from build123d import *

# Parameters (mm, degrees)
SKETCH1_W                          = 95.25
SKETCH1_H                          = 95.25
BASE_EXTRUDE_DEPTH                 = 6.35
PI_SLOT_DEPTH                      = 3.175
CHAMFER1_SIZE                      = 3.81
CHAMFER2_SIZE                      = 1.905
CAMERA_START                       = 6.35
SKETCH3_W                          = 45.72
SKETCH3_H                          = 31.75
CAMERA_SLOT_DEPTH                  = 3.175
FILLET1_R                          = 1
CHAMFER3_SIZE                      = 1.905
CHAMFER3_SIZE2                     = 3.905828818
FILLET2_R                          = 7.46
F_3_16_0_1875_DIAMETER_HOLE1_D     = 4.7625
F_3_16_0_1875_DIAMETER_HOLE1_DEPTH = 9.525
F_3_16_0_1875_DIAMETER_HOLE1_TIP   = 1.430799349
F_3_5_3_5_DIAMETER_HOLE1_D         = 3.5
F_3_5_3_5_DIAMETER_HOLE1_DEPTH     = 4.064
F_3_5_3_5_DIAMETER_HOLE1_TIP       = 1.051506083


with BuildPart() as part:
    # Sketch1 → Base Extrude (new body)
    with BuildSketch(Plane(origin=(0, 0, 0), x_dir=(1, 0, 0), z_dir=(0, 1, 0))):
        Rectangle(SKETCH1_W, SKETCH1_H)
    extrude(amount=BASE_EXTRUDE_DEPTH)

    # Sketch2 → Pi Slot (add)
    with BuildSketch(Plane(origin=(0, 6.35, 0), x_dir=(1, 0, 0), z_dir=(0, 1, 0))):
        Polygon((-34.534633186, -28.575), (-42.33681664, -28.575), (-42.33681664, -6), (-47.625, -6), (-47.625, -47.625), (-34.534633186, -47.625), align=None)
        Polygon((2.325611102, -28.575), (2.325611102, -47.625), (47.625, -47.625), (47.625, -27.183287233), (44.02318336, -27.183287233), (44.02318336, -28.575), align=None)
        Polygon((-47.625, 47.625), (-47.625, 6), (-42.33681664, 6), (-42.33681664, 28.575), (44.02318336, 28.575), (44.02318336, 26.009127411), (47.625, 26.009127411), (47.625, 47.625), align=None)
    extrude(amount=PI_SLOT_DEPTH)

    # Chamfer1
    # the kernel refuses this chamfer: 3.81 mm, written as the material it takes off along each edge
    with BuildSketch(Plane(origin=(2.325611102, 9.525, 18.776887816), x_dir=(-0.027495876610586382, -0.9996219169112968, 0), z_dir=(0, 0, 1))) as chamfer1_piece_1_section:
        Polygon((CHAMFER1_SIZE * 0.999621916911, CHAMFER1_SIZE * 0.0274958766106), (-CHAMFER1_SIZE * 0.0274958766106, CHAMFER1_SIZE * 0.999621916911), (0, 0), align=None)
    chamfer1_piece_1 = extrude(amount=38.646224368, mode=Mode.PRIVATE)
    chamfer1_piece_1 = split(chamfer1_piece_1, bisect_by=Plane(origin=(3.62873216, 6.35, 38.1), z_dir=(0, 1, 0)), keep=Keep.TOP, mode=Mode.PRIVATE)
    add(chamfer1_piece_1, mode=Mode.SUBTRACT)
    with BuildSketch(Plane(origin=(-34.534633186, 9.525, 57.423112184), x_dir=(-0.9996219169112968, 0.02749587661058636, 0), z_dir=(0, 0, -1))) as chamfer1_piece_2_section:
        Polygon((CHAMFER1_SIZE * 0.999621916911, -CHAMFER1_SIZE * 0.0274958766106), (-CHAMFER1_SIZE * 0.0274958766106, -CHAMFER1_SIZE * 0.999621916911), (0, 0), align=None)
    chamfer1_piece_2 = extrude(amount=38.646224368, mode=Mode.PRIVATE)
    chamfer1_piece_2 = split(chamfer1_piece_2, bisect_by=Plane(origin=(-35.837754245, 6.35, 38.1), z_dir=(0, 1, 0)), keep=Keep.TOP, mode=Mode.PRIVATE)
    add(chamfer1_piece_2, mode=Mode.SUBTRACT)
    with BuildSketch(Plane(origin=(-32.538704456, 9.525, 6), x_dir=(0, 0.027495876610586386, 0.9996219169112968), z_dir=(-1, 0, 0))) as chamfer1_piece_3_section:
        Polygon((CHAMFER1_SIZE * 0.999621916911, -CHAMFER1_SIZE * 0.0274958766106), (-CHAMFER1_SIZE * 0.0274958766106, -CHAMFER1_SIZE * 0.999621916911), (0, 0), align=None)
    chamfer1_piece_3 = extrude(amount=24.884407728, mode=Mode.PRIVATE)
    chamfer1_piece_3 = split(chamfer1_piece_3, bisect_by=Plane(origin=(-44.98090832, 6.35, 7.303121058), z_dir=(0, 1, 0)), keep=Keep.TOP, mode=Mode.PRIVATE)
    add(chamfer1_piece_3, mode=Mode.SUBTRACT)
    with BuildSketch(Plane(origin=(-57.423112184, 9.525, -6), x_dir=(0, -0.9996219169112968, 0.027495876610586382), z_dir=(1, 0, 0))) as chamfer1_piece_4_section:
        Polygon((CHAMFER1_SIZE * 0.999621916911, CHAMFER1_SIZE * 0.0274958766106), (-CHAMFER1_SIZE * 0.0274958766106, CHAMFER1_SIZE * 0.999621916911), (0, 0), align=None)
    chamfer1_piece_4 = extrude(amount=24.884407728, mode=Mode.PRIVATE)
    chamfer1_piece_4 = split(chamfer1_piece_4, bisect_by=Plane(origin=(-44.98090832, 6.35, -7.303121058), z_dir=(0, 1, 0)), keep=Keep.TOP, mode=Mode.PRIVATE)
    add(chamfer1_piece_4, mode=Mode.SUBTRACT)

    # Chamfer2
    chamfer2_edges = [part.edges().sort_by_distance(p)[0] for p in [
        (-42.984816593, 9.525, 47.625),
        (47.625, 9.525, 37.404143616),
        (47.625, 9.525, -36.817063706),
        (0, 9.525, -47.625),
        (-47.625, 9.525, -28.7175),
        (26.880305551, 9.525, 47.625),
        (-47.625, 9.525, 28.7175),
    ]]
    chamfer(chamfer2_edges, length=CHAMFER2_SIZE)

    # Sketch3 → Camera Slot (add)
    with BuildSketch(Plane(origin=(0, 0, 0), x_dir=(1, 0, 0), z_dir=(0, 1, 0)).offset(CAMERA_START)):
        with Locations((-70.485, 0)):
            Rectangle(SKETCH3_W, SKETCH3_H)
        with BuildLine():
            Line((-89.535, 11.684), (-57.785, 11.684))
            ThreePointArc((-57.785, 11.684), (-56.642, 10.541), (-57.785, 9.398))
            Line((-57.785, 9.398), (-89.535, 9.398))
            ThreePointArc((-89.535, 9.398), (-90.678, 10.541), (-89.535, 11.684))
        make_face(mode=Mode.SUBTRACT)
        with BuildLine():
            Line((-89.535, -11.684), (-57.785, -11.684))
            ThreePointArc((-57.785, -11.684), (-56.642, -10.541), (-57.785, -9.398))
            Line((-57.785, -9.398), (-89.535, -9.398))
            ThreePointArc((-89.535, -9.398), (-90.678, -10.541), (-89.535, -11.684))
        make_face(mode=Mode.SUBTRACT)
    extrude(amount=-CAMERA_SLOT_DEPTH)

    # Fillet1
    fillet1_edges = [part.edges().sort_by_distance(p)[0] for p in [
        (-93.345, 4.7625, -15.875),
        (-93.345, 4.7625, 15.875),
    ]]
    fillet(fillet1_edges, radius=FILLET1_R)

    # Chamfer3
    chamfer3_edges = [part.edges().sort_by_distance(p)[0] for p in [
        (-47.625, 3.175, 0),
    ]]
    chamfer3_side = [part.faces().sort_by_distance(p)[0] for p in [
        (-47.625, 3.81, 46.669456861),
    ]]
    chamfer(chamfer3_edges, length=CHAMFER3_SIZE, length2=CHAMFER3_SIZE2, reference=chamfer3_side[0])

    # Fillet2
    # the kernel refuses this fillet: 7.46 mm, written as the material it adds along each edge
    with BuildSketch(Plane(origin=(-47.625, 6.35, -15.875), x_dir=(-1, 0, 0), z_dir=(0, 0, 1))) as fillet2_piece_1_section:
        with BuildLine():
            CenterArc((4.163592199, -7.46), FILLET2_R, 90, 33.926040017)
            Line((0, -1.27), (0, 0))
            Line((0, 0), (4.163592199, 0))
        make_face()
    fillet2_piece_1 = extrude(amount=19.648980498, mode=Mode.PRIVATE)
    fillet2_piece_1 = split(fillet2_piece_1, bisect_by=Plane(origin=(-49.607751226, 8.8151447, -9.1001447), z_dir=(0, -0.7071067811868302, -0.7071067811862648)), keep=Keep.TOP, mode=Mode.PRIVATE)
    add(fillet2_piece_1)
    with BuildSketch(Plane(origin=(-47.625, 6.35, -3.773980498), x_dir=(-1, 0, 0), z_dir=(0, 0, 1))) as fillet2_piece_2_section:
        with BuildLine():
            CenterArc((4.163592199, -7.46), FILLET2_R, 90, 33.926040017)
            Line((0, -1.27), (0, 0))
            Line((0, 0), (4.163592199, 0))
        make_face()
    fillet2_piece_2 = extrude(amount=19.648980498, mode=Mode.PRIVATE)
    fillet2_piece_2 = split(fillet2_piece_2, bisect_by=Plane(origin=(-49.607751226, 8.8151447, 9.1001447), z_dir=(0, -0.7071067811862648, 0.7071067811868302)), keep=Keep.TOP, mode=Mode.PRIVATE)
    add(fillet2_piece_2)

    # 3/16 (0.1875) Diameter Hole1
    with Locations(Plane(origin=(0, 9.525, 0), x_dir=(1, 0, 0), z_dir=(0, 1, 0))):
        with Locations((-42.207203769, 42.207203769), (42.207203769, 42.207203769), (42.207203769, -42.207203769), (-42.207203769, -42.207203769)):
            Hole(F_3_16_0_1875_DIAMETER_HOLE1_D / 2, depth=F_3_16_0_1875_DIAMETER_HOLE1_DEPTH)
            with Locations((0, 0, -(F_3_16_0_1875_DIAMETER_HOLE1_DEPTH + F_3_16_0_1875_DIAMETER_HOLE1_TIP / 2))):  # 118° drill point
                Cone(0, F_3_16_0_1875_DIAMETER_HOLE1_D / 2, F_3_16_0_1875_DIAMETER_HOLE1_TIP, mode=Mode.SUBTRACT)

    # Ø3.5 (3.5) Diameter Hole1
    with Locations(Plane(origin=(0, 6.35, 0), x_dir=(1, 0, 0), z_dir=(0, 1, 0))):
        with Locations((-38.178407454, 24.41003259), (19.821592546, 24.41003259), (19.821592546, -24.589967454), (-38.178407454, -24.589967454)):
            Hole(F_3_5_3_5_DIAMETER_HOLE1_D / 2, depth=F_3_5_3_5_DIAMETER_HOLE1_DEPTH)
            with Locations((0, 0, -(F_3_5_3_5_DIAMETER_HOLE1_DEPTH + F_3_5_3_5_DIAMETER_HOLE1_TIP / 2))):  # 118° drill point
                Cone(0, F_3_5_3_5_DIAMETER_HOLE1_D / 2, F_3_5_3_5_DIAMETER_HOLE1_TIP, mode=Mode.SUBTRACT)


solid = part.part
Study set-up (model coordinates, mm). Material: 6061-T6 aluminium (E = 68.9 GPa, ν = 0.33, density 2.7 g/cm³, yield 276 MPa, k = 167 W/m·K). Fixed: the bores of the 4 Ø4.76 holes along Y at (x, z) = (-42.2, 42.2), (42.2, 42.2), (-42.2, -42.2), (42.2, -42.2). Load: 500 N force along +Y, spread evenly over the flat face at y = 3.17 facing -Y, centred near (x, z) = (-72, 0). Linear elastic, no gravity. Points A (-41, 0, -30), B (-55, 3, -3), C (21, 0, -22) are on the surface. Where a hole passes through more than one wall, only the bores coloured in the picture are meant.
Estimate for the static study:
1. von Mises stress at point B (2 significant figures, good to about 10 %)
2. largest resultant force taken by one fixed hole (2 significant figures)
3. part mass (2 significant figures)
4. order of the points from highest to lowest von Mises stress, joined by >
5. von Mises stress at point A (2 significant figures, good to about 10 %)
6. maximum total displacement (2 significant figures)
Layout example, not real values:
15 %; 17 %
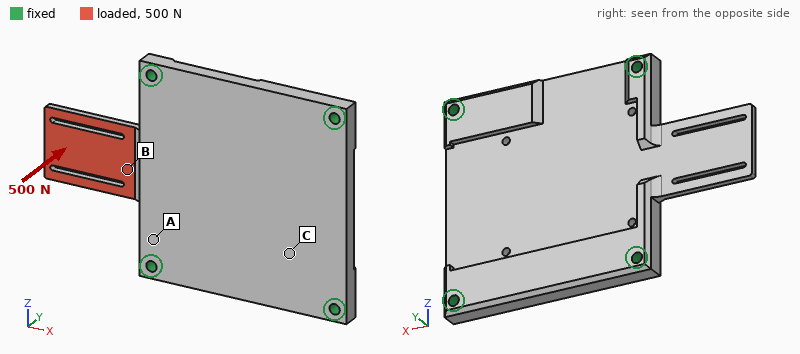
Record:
160 MPa; 440 N; 190 g; B > A > C; 32 MPa; 1.3 mm
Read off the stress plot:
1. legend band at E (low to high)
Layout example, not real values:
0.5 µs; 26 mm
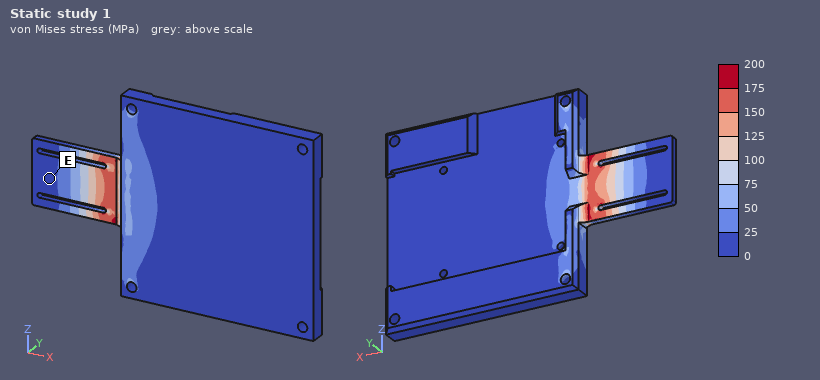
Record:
0 to 25 MPa
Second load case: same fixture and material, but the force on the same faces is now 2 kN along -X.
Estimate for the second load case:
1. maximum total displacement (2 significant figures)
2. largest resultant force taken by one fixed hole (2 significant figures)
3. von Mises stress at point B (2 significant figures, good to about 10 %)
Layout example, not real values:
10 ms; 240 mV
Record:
0.39 mm; 570 N; 70 MPa
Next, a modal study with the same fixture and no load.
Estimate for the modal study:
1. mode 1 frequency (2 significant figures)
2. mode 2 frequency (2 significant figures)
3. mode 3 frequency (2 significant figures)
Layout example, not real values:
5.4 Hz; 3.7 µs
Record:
1200 Hz; 3600 Hz; 3800 Hz
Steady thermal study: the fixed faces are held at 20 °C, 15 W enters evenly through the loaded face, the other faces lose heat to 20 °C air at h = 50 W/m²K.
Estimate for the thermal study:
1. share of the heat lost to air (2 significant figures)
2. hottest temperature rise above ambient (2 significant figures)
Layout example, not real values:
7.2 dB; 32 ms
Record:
26 %; 27 K
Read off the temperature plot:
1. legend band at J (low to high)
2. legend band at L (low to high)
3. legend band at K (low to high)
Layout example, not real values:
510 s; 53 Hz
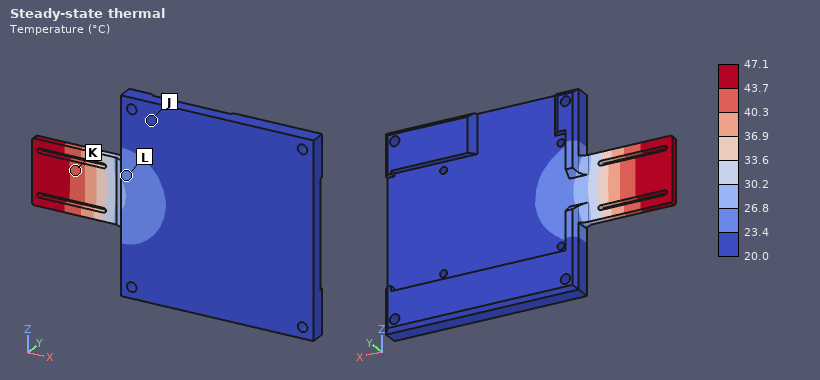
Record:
20.0 to 23.4 °C; 23.4 to 26.8 °C; 40.3 to 43.7 °C
